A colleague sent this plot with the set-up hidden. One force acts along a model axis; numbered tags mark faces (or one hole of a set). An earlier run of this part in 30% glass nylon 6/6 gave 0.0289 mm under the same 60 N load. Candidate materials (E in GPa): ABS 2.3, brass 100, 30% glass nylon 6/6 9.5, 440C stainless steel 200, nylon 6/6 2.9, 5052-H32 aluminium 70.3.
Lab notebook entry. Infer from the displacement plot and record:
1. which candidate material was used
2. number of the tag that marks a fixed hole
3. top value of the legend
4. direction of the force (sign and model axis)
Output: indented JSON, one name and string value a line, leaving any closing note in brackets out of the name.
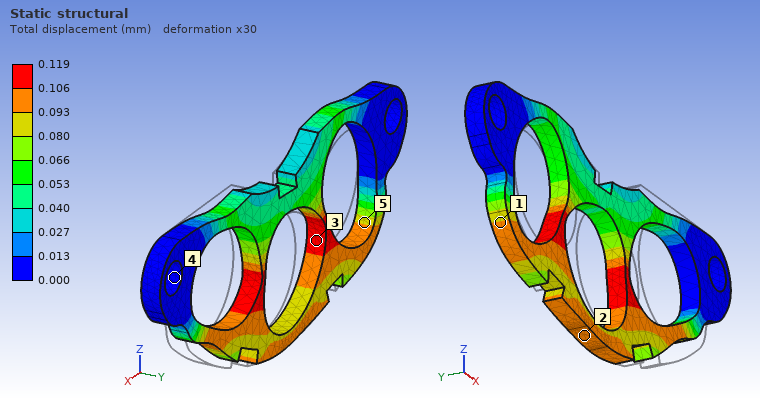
{
  "which candidate material was used": "ABS",
  "number of the tag that marks a fixed hole": "4",
  "top value of the legend": "0.119 mm",
  "direction of the force": "-X"
}
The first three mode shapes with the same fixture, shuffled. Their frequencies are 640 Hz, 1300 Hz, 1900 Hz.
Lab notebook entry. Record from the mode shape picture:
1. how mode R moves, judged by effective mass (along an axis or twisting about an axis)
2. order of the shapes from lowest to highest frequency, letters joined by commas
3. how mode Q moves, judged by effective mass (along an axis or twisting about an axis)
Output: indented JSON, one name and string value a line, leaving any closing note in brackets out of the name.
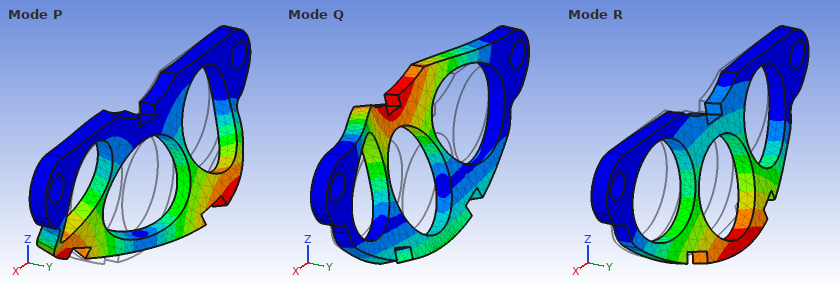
{
  "how mode R moves, judged by effective mass": "along Y",
  "order of the shapes from lowest to highest frequency, letters joined by commas": "R, Q, P",
  "how mode Q moves, judged by effective mass": "along Y"
}
